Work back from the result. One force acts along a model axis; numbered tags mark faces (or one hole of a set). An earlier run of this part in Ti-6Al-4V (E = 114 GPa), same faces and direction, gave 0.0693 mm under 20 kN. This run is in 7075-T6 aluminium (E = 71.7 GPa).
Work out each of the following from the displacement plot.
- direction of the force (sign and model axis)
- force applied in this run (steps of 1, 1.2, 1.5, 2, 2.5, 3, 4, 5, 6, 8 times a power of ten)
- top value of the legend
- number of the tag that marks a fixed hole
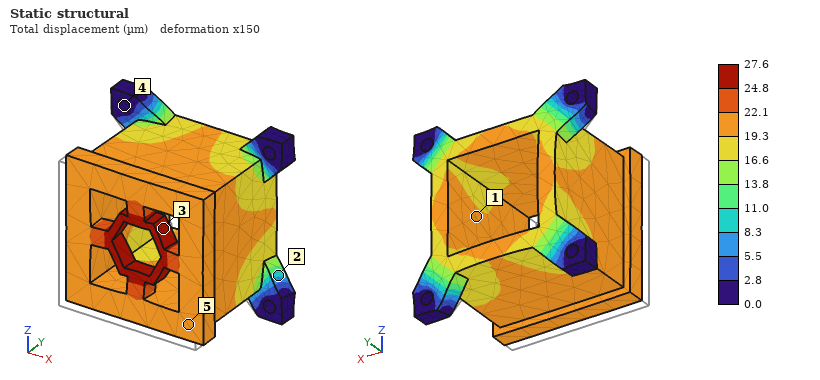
+Y
5 kN
27.6 µm
4
